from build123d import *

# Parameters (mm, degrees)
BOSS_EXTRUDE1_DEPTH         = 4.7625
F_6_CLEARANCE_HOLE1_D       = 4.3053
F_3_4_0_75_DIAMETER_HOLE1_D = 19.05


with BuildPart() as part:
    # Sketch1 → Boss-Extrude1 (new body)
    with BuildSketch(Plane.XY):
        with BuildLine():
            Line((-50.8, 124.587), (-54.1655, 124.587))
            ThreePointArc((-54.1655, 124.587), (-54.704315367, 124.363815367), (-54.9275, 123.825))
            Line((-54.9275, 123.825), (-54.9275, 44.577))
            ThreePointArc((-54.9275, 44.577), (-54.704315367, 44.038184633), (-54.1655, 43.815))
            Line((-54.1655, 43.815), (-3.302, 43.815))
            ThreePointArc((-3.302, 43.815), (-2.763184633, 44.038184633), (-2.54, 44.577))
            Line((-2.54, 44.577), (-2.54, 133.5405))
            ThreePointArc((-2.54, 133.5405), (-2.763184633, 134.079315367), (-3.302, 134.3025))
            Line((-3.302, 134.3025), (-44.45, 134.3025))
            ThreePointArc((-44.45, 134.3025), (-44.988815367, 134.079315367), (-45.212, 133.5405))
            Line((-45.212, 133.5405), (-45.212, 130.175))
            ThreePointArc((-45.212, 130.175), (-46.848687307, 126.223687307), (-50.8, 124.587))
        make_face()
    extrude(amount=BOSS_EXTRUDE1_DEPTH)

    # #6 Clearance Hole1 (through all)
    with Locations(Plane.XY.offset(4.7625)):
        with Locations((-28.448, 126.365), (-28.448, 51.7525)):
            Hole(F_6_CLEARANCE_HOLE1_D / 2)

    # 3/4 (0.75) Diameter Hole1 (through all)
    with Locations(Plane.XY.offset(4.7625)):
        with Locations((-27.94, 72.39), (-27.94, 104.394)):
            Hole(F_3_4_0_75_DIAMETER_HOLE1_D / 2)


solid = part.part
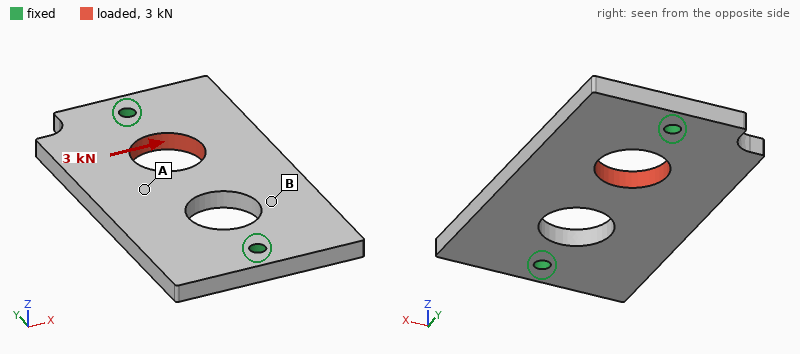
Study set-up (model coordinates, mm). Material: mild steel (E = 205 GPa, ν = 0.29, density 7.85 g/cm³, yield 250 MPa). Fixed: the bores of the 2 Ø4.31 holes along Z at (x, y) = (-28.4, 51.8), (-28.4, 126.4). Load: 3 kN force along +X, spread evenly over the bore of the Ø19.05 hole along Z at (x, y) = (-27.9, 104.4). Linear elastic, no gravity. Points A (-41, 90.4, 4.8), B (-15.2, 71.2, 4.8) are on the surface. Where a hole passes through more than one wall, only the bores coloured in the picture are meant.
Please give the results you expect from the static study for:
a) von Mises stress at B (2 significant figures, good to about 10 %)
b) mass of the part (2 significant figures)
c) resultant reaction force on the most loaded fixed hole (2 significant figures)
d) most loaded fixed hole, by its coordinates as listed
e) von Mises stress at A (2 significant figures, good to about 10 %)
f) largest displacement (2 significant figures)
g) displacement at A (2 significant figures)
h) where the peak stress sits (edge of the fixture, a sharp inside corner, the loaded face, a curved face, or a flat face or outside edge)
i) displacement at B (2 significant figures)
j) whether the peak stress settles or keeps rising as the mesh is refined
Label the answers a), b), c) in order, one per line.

a) 14 MPa
b) 150 g
c) 2.1 kN
d) (-28.4, 126.4)
e) 6.1 MPa
f) 5.9 µm
g) 5.4 µm
h) edge of the fixture
i) 2.9 µm
j) keeps rising
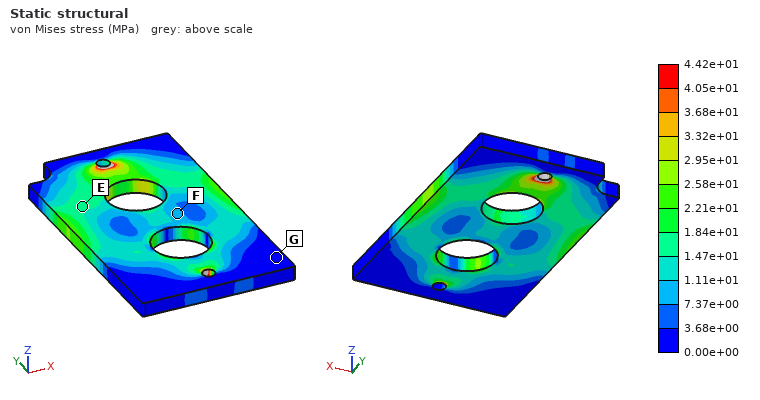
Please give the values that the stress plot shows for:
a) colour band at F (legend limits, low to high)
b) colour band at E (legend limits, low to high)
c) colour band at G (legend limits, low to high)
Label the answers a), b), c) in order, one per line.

a) 7.37e+00 to 1.11e+01 MPa
b) 1.47e+01 to 1.84e+01 MPa
c) 0.00e+00 to 3.68e+00 MPa
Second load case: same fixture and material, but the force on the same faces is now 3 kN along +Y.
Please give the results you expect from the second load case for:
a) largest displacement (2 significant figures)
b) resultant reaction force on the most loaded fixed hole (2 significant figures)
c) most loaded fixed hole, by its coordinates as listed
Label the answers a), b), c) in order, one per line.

a) 4.2 µm
b) 2.0 kN
c) (-28.4, 126.4)
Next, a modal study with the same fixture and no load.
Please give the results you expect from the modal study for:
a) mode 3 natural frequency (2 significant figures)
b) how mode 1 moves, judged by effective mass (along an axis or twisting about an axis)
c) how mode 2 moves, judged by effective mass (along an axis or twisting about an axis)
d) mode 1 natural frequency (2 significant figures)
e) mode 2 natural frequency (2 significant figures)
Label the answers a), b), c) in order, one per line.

a) 5800 Hz
b) twisting about Y
c) along Z
d) 2800 Hz
e) 3100 Hz
